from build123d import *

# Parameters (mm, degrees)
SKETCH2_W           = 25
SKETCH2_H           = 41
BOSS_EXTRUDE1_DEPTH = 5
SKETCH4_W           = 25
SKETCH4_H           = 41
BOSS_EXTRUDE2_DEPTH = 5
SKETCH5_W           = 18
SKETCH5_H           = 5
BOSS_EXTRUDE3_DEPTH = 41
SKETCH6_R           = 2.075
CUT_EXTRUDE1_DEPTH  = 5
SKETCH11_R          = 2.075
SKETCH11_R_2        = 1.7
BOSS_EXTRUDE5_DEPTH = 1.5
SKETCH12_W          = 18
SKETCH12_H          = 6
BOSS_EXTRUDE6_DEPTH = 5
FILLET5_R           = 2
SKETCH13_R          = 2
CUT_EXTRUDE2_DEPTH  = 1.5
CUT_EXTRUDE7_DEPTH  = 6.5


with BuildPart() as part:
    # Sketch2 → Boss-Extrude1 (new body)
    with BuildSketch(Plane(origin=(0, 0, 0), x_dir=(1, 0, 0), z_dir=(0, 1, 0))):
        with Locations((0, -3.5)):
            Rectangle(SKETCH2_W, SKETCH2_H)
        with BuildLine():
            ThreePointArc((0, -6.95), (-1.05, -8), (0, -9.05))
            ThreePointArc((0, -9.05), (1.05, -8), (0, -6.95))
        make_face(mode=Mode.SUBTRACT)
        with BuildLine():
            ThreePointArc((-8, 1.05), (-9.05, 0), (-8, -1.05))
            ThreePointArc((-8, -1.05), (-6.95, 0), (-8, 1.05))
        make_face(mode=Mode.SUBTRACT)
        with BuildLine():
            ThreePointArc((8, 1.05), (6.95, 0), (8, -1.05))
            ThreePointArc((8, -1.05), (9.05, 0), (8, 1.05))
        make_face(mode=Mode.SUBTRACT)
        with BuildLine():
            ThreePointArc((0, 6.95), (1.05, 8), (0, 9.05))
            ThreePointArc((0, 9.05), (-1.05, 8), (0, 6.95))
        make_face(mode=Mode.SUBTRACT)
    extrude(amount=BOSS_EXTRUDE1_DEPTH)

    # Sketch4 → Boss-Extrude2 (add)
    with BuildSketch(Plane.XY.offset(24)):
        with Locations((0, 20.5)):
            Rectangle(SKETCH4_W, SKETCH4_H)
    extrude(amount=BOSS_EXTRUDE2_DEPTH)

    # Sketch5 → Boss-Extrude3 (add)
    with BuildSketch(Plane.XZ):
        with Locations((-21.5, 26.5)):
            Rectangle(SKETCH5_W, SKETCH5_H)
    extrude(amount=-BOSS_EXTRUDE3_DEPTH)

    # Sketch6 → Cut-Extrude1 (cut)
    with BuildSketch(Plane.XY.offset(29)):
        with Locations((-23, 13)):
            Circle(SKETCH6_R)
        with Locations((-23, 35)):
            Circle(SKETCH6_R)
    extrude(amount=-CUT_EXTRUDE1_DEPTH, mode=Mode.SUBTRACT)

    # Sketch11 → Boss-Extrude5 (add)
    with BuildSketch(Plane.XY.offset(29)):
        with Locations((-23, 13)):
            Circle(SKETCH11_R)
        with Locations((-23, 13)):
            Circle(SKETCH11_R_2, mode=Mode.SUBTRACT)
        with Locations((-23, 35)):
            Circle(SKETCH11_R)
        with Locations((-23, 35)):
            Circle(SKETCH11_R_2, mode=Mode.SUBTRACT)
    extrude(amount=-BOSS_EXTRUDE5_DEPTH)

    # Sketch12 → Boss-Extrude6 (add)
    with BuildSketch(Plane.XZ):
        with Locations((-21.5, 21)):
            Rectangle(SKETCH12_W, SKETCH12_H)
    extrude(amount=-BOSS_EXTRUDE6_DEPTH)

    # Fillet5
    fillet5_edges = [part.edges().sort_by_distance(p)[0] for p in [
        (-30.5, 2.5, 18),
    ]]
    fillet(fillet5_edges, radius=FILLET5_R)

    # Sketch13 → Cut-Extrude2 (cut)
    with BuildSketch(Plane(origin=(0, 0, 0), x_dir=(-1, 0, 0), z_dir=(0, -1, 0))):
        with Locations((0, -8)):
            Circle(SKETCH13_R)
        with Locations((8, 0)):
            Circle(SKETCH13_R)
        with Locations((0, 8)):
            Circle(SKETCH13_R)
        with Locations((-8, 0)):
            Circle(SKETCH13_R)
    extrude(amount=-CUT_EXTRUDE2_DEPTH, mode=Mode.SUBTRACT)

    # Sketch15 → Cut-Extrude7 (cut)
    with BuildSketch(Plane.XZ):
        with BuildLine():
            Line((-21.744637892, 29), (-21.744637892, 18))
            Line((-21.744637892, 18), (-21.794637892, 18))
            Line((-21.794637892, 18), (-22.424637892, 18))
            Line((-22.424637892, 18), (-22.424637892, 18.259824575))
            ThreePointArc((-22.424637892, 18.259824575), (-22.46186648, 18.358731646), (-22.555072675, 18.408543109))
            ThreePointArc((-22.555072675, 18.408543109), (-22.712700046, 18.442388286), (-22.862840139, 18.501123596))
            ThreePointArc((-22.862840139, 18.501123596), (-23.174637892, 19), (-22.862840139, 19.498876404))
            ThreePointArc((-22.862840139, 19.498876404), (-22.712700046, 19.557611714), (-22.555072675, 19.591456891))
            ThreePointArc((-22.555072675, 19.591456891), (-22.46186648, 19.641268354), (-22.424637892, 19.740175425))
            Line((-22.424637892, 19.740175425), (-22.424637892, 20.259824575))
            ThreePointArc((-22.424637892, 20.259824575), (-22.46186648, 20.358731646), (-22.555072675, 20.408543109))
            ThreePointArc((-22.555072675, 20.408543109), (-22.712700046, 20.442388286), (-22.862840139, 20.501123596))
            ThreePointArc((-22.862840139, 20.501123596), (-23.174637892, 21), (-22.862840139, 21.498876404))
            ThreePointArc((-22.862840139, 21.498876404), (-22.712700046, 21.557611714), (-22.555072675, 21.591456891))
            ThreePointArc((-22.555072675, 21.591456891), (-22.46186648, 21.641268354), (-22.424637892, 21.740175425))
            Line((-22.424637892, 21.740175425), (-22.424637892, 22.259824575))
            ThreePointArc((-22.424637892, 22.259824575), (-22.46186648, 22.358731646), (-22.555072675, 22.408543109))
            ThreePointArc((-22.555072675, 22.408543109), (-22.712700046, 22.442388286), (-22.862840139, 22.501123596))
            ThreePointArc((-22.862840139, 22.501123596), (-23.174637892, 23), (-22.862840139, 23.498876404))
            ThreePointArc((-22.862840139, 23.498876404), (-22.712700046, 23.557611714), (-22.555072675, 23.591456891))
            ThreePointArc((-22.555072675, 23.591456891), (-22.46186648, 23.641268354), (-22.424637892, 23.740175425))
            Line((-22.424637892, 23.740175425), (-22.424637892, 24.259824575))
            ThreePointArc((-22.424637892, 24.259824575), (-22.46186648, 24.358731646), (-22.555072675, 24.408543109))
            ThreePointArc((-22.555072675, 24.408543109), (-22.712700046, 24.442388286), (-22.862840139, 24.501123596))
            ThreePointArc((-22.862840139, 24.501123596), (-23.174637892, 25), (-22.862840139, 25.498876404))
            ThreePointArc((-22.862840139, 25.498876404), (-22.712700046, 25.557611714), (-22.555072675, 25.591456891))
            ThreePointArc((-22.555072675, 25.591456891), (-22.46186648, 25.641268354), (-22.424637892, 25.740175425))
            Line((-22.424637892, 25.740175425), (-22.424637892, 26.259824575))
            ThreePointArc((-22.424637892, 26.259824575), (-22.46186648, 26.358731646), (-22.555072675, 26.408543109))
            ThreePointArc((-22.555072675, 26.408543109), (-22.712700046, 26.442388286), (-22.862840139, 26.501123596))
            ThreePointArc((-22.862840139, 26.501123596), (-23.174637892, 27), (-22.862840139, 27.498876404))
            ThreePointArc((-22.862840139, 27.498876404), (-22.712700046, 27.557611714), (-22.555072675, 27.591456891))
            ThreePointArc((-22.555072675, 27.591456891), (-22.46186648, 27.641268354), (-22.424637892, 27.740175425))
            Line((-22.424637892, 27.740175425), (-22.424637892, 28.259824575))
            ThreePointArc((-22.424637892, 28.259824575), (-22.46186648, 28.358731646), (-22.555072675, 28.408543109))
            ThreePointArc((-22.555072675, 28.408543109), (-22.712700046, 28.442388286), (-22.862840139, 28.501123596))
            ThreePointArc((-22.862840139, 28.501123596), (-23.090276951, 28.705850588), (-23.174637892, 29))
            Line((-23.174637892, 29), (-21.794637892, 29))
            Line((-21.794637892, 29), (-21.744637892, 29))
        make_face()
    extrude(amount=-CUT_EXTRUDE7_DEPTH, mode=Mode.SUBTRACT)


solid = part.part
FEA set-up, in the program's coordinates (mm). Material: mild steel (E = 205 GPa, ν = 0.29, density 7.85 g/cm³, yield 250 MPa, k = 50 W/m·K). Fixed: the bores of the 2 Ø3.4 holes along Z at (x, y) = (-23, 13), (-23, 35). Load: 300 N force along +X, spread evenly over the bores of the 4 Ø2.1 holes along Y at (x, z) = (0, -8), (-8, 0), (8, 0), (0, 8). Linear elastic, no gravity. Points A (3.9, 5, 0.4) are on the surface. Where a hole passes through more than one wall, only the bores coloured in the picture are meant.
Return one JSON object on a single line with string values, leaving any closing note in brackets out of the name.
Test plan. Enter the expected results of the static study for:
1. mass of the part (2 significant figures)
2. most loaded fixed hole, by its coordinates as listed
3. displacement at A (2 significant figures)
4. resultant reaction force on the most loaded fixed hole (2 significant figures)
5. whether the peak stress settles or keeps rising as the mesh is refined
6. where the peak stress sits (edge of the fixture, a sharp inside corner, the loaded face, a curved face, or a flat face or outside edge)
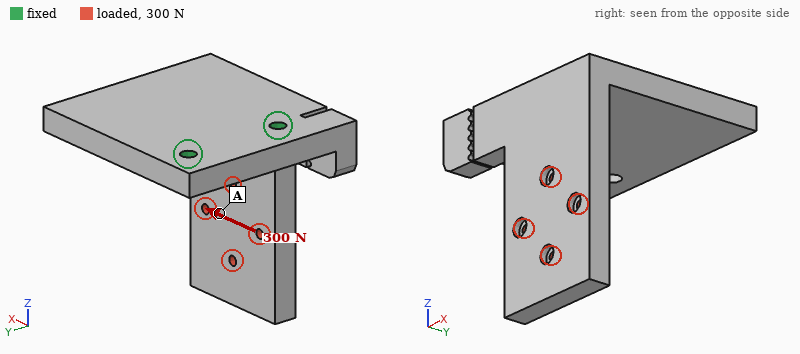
{"mass of the part": "110 g", "most loaded fixed hole, by its coordinates as listed": "(-23, 13)", "displacement at A": "0.13 mm", "resultant reaction force on the most loaded fixed hole": "440 N", "whether the peak stress settles or keeps rising as the mesh is refined": "keeps rising", "where the peak stress sits": "edge of the fixture"}
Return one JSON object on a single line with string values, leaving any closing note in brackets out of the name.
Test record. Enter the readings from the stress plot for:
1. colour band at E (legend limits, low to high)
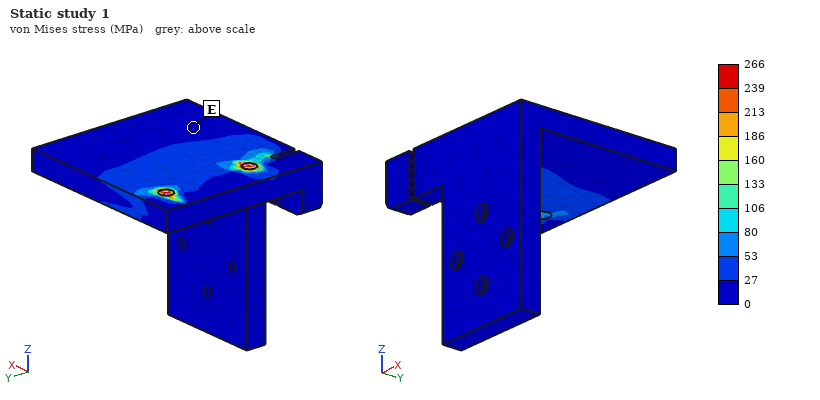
{"colour band at E": "0 to 27 MPa"}
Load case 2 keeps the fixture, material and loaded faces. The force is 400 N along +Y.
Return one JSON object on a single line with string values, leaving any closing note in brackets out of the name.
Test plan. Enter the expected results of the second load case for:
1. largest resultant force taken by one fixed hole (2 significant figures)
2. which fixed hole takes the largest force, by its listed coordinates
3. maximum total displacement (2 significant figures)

{"largest resultant force taken by one fixed hole": "870 N", "which fixed hole takes the largest force, by its listed coordinates": "(-23, 35)", "maximum total displacement": "0.22 mm"}
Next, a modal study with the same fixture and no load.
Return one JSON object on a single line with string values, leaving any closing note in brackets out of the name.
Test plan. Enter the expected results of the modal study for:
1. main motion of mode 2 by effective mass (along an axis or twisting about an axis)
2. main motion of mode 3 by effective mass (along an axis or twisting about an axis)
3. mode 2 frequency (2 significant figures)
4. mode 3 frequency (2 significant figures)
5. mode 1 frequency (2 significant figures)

{"main motion of mode 2 by effective mass": "along Y", "main motion of mode 3 by effective mass": "along Z", "mode 2 frequency": "1500 Hz", "mode 3 frequency": "4600 Hz", "mode 1 frequency": "950 Hz"}
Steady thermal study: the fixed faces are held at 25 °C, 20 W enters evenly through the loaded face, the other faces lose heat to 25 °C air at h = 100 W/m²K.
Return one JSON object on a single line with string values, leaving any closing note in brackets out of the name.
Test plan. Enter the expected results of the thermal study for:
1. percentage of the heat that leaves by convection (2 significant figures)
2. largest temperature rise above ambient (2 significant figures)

{"percentage of the heat that leaves by convection": "79 %", "largest temperature rise above ambient": "61 K"}
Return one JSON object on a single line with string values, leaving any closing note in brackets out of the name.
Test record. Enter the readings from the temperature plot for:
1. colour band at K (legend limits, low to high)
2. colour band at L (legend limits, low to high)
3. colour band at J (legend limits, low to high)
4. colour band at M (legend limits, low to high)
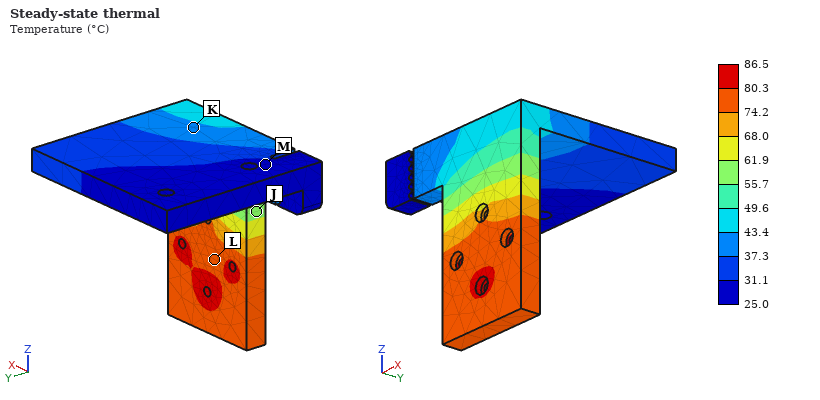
{"colour band at K": "37.3 to 43.4 °C", "colour band at L": "74.2 to 80.3 °C", "colour band at J": "55.7 to 61.9 °C", "colour band at M": "25.0 to 31.1 °C"}
